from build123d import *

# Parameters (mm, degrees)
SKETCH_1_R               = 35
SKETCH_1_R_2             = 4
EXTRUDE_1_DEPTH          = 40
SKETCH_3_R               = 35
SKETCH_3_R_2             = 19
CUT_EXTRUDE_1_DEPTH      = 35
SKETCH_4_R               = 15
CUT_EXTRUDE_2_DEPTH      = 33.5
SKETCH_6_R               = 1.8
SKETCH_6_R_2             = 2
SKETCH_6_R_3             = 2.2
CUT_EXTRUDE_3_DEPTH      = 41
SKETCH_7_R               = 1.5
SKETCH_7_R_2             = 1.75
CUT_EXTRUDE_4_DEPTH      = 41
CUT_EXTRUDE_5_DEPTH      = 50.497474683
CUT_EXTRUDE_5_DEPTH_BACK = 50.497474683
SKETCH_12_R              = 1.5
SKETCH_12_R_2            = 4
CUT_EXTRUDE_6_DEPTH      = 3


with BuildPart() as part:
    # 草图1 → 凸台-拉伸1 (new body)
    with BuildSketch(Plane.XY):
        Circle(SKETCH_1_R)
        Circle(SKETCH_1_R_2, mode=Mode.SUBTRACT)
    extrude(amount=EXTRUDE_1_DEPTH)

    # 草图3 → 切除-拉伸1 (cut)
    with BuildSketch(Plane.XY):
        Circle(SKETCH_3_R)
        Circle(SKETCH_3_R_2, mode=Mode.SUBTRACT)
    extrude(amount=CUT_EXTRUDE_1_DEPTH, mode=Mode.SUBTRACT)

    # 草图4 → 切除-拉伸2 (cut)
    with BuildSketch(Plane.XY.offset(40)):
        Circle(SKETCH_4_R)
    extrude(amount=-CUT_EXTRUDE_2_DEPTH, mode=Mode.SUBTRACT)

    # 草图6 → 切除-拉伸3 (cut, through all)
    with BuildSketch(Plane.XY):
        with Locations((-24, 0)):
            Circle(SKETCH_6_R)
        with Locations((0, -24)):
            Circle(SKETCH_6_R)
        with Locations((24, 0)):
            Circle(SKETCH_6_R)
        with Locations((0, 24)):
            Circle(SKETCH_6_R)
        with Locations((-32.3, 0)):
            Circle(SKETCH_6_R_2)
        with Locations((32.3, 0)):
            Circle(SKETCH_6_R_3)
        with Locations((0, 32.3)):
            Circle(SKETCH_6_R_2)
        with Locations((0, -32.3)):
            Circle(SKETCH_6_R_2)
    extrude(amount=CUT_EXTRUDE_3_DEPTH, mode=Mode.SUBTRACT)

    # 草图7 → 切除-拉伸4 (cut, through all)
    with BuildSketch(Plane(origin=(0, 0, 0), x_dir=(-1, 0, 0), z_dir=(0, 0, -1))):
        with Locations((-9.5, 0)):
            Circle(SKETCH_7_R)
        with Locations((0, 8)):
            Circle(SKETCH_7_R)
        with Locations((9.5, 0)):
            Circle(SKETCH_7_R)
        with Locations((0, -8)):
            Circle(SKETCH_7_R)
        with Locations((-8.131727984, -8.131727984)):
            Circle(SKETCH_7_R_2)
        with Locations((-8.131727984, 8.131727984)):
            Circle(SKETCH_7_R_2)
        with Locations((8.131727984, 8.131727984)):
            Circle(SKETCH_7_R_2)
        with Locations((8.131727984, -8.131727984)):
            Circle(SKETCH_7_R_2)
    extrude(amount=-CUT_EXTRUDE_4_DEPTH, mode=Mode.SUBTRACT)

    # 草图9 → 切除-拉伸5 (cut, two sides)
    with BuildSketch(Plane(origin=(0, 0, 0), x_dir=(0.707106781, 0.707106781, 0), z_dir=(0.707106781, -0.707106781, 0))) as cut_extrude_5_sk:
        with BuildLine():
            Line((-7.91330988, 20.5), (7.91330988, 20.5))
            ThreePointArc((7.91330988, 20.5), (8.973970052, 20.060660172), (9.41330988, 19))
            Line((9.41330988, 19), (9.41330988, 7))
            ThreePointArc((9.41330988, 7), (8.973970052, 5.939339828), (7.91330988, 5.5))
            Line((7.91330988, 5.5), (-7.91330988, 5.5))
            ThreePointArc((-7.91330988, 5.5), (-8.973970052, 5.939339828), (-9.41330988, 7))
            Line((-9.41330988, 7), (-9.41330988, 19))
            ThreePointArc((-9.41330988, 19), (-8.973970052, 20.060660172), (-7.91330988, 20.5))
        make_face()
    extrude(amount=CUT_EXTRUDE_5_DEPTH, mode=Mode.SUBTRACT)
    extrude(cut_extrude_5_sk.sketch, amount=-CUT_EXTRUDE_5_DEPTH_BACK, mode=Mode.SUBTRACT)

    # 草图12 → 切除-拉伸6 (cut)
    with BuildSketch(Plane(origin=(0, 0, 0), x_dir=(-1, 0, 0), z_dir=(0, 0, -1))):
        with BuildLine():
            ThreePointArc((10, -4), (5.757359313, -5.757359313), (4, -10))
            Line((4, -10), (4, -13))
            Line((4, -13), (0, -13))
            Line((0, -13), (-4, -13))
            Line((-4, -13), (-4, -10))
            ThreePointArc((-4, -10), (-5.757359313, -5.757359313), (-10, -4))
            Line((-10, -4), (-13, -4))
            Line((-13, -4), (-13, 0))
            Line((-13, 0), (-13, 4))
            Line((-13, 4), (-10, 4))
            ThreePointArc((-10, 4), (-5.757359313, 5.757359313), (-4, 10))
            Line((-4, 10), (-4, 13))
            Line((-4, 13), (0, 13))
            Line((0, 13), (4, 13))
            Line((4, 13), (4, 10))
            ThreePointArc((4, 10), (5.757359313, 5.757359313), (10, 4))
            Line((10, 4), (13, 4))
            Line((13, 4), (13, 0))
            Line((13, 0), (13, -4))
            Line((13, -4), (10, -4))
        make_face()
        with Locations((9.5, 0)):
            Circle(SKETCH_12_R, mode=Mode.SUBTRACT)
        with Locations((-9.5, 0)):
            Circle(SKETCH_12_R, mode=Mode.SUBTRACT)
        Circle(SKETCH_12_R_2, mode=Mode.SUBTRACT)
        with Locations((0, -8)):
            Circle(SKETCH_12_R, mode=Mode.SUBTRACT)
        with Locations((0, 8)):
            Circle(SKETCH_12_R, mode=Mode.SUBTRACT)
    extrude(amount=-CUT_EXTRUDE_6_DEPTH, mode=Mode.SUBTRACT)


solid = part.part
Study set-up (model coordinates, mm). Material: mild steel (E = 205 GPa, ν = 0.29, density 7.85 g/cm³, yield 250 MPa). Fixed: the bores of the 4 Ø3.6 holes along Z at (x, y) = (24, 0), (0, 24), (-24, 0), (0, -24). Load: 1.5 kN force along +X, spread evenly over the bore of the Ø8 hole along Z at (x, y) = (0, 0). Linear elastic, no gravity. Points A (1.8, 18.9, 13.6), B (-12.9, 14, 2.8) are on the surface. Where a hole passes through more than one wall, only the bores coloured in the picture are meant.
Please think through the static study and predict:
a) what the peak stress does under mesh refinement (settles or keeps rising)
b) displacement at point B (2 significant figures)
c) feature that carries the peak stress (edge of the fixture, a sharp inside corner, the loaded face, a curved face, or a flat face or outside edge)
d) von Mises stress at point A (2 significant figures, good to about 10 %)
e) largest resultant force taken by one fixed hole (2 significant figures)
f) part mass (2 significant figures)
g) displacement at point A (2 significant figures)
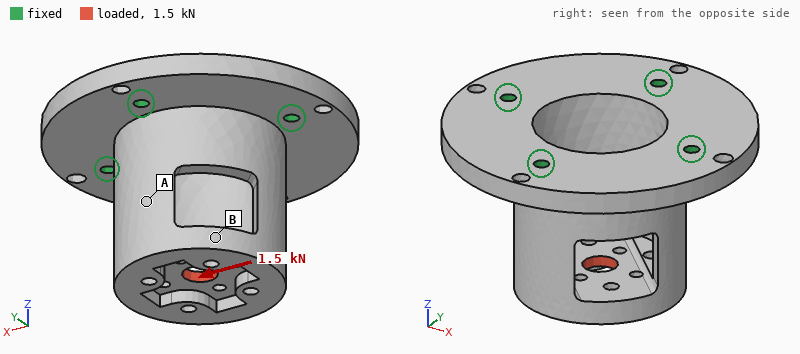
keeps rising
17 µm
edge of the fixture
28 MPa
1.2 kN
240 g
8.8 µm
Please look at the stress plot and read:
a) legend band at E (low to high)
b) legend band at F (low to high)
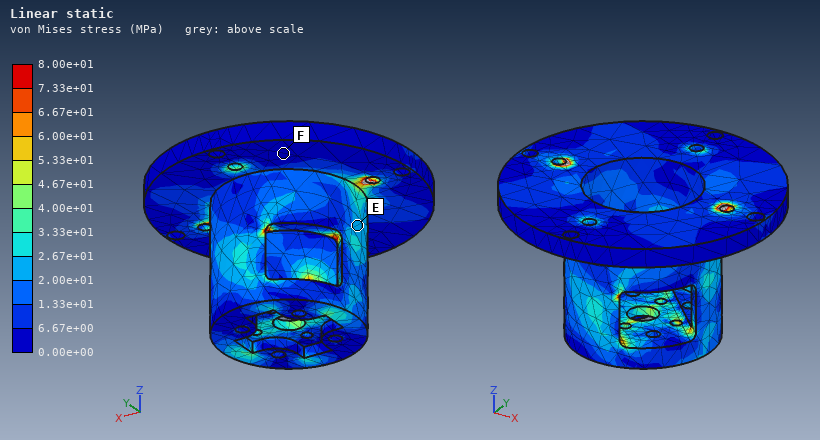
2.00e+01 to 2.67e+01 MPa
0.00e+00 to 6.67e+00 MPa
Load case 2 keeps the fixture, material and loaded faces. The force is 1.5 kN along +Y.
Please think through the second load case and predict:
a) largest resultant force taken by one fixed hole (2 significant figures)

1.2 kN
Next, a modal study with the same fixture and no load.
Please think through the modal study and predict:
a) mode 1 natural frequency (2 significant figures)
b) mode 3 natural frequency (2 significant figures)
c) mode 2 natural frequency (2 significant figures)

5700 Hz
11 kHz
7500 Hz
